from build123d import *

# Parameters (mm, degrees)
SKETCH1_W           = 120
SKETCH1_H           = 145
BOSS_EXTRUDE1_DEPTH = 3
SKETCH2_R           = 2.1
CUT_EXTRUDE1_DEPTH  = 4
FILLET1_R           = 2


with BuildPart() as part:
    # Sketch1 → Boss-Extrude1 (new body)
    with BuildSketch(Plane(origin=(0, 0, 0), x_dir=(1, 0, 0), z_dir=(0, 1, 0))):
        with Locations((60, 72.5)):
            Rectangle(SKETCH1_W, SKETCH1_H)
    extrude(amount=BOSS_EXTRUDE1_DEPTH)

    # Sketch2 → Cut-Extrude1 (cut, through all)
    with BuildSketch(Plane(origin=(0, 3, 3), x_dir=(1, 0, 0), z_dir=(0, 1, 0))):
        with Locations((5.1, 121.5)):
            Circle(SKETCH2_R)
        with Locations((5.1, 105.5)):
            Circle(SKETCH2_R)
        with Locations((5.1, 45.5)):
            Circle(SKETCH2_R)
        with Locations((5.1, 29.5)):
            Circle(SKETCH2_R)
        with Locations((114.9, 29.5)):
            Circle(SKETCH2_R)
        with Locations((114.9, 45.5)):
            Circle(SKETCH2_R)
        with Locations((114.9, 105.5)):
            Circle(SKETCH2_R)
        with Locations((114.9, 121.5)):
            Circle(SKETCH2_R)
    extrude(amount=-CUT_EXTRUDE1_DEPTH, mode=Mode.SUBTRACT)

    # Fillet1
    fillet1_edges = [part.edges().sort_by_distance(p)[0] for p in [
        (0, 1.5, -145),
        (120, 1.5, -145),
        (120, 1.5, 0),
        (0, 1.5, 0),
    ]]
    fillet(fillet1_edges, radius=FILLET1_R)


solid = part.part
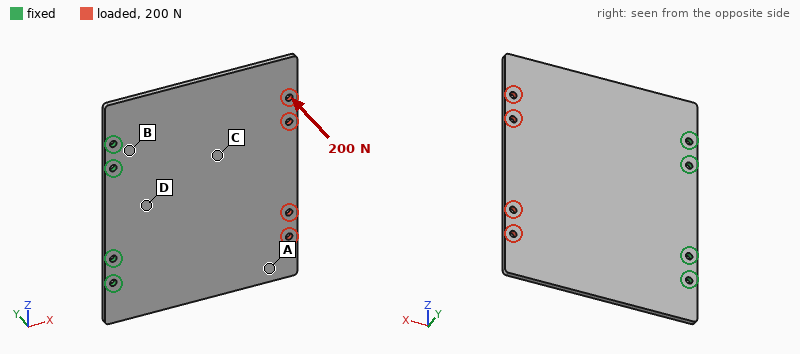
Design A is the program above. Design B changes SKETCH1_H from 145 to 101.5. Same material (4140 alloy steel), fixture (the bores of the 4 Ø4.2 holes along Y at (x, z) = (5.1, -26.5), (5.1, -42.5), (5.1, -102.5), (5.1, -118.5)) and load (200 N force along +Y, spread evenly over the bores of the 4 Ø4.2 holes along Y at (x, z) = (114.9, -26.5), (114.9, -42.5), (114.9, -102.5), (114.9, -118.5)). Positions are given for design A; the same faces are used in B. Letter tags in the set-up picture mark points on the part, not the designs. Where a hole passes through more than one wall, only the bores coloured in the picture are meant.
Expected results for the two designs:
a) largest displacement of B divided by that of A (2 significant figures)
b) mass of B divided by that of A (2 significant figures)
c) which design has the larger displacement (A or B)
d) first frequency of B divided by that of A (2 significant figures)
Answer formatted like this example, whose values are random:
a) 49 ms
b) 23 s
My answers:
a) 1.4
b) 0.70
c) B
d) 1.0
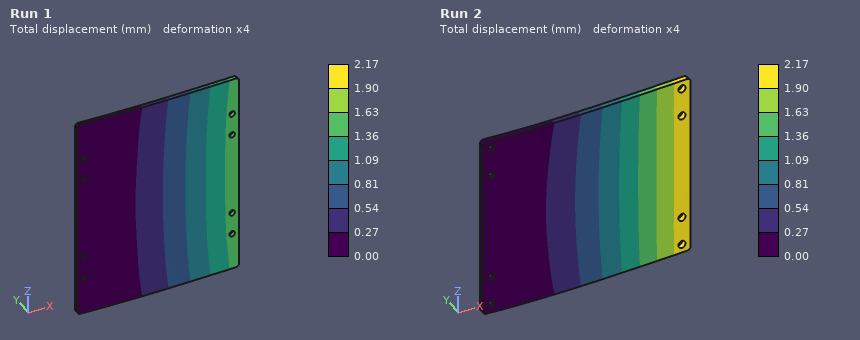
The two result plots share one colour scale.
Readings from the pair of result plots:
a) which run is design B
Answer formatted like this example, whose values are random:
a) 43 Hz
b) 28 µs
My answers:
a) Run 2
